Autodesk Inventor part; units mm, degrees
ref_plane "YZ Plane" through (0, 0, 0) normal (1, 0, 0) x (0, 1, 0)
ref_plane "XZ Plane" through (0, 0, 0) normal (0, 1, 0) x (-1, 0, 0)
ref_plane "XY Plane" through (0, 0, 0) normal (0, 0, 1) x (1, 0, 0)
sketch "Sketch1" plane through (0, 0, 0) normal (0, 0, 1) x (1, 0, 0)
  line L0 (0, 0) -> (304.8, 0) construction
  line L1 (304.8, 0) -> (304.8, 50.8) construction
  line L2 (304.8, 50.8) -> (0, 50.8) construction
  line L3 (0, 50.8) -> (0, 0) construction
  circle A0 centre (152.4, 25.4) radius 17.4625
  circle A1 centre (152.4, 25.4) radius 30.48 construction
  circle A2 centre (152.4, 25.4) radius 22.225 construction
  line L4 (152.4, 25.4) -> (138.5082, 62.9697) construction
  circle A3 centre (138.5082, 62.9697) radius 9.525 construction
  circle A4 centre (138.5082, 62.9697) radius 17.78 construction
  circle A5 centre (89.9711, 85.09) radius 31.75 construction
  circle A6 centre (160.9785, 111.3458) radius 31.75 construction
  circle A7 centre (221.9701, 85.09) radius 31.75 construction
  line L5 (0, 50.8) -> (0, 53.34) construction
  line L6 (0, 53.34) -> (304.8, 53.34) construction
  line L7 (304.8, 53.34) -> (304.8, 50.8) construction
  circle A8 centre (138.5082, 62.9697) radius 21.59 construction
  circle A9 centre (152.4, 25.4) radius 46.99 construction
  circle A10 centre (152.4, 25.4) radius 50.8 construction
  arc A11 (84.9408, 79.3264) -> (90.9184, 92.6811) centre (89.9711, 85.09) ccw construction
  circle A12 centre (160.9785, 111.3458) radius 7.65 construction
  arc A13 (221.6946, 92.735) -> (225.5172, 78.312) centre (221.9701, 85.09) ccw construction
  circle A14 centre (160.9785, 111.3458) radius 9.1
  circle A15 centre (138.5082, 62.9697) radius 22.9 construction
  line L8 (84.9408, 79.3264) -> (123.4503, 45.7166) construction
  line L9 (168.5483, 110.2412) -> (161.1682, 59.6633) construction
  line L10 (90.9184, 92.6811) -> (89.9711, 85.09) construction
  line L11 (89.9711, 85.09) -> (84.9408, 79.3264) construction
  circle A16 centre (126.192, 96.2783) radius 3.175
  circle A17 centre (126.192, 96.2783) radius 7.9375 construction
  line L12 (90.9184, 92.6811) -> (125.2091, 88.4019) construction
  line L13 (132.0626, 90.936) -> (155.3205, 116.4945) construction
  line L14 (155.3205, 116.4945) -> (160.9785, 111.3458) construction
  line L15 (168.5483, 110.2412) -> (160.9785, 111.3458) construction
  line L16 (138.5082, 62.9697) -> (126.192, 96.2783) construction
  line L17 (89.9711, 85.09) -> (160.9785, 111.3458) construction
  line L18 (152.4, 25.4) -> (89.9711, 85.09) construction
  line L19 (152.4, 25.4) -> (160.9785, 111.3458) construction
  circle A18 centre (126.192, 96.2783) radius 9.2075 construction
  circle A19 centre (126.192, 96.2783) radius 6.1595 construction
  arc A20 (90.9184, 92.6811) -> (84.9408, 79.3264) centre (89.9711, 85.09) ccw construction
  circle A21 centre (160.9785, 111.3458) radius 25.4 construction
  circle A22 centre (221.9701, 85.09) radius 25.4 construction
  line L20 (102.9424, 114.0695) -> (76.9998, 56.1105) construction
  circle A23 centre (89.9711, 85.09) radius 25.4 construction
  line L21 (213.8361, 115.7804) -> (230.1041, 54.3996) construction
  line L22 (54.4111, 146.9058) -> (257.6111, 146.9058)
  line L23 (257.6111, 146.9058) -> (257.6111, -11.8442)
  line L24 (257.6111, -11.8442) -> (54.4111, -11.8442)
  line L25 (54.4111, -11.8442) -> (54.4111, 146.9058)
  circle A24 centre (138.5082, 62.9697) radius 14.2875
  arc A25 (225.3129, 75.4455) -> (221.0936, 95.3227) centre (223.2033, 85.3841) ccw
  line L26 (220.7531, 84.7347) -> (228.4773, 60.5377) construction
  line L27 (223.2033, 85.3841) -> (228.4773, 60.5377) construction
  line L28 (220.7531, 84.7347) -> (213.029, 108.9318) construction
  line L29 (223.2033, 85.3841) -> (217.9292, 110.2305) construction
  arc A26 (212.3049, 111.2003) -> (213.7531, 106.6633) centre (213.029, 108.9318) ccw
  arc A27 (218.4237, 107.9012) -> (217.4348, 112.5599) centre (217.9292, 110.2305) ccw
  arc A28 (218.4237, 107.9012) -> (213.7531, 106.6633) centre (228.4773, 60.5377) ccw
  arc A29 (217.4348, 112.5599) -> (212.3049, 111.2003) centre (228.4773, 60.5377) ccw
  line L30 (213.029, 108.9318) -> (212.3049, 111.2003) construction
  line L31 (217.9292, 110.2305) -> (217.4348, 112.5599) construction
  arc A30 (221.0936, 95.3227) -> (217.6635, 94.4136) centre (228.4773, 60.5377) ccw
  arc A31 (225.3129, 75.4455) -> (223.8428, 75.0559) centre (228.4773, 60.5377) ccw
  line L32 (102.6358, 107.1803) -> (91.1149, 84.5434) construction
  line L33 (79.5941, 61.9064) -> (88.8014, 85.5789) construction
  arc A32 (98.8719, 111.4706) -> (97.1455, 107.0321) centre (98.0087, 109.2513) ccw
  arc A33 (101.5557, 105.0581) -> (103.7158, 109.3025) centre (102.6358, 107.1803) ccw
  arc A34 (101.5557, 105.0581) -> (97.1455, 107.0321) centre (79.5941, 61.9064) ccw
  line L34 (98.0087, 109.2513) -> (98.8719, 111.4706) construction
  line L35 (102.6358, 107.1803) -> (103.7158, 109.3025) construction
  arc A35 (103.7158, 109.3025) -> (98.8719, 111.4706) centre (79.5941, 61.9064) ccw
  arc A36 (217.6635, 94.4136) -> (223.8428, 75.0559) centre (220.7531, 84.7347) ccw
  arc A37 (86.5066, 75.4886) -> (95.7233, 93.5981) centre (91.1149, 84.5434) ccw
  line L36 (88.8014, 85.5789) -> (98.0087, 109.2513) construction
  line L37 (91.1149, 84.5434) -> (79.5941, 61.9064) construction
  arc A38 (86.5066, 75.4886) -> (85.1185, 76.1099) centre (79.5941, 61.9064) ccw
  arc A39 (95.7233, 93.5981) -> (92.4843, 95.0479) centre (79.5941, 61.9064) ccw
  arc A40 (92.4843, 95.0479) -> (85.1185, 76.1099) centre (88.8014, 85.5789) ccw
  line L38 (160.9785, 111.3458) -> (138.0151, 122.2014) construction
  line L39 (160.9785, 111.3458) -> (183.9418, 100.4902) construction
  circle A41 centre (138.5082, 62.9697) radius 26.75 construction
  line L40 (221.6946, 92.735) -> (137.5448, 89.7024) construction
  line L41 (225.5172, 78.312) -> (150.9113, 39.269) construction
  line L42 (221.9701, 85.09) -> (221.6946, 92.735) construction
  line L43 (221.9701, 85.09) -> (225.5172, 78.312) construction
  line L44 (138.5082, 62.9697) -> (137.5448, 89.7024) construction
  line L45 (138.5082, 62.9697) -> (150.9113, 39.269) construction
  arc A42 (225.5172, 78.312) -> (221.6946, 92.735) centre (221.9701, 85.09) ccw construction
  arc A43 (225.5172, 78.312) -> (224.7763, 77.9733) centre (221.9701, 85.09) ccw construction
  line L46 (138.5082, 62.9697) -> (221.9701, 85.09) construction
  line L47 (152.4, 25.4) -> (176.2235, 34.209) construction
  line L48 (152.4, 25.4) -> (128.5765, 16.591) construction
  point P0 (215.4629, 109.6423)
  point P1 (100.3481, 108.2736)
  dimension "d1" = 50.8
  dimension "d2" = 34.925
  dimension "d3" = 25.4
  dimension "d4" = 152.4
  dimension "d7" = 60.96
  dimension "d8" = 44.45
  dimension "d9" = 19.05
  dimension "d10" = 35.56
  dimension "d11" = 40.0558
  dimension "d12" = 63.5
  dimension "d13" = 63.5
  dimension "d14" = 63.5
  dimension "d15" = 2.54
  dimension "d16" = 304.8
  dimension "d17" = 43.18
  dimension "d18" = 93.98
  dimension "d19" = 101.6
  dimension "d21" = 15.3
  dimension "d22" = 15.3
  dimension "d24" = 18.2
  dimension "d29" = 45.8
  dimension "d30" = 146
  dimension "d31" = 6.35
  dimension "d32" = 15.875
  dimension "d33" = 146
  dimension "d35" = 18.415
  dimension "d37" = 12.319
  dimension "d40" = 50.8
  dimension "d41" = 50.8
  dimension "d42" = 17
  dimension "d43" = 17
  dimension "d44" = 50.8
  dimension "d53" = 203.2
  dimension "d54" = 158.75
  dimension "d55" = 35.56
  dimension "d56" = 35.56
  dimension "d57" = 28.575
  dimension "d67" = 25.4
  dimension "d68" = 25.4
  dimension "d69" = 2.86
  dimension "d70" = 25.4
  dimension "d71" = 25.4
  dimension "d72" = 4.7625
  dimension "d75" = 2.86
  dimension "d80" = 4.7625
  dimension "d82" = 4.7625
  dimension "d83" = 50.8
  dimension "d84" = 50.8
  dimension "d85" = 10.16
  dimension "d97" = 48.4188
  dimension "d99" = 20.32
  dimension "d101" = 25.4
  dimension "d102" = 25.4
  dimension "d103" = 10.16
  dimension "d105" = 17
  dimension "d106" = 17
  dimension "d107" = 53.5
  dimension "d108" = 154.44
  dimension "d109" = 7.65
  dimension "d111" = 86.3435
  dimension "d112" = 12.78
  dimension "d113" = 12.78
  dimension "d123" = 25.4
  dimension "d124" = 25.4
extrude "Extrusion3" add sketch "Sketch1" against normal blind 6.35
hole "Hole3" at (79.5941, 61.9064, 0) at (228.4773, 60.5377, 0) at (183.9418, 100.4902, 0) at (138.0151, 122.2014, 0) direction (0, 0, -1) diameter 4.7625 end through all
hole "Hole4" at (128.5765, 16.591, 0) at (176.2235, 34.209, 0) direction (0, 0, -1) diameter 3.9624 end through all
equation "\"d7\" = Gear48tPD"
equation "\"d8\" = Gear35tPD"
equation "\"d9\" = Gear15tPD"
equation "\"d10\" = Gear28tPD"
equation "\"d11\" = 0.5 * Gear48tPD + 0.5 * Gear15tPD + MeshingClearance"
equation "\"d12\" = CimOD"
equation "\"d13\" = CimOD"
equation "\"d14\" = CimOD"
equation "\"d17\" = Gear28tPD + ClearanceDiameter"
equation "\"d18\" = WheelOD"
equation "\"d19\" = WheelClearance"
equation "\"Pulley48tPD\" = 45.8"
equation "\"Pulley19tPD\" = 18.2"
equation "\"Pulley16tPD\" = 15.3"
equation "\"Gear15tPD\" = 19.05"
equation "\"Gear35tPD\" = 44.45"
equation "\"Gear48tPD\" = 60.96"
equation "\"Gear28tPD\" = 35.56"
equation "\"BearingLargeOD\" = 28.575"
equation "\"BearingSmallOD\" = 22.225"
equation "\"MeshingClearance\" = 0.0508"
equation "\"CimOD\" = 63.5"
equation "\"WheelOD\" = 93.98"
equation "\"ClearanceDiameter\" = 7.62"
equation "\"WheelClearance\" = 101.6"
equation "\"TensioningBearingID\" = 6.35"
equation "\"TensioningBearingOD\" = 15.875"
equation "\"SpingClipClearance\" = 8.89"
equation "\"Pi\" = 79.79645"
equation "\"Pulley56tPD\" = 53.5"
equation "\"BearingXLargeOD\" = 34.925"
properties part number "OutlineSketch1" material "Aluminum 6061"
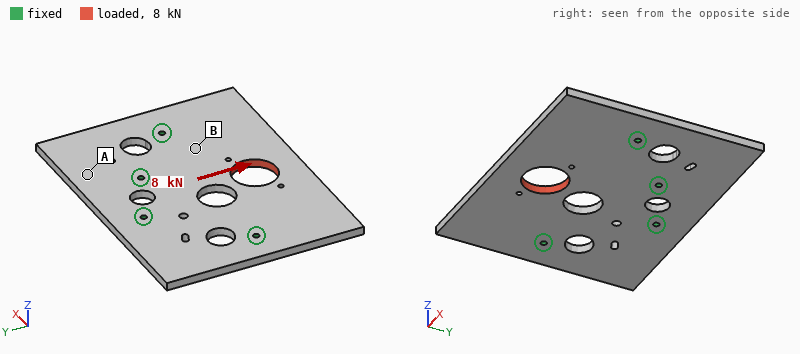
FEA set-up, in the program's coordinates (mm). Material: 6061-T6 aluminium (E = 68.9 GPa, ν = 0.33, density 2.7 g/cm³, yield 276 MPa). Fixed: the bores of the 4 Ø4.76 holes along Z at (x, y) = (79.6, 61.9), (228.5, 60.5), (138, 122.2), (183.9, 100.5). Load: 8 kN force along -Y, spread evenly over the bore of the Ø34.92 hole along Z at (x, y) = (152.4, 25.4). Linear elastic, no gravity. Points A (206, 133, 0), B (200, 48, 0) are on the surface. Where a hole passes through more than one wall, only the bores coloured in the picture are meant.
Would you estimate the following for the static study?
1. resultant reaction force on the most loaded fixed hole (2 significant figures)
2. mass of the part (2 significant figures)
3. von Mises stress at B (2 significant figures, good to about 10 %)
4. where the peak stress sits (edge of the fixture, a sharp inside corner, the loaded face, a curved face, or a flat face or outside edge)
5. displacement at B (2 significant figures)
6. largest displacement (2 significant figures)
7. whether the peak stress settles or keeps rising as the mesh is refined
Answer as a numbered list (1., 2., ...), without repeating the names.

1. 2.7 kN
2. 500 g
3. 7.7 MPa
4. edge of the fixture
5. 6.5 µm
6. 27 µm
7. keeps rising
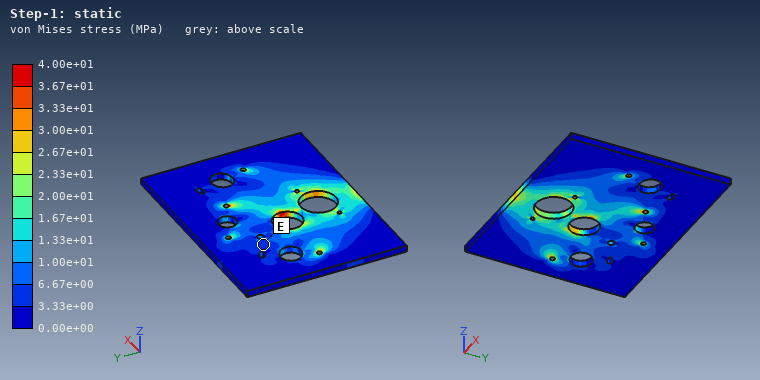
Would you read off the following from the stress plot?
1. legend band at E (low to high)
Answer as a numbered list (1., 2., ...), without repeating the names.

1. 3.33e+00 to 6.67e+00 MPa
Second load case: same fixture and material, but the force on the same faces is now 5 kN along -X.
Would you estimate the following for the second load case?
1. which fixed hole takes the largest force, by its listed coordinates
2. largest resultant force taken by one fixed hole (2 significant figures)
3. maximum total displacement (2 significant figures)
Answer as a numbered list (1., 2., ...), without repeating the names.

1. (228.5, 60.5)
2. 2.7 kN
3. 20 µm
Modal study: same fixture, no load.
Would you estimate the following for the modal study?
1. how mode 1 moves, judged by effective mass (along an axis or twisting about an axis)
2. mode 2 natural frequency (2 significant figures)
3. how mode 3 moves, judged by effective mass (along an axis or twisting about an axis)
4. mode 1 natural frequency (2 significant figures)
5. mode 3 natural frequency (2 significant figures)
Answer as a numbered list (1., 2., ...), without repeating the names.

1. along Z
2. 1100 Hz
3. along Z
4. 680 Hz
5. 1200 Hz
